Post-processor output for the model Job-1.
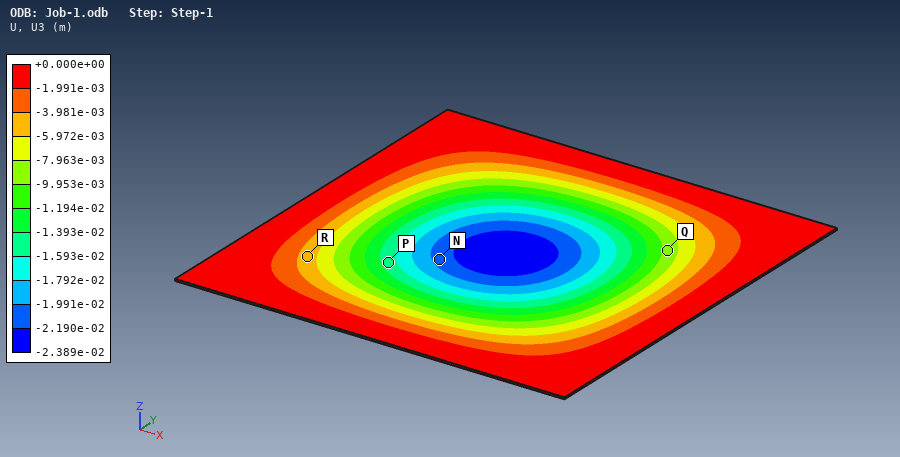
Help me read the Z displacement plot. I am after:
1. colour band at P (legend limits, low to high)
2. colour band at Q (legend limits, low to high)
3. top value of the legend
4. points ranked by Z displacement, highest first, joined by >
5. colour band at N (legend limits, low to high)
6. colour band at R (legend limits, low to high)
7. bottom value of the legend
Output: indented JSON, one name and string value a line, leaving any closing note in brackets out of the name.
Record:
{
  "colour band at P": "-1.593e-02 to -1.393e-02 m",
  "colour band at Q": "-9.953e-03 to -7.963e-03 m",
  "top value of the legend": "+0.000e+00 m",
  "points ranked by Z displacement, highest first, joined by >": "R > Q > P > N",
  "colour band at N": "-2.190e-02 to -1.991e-02 m",
  "colour band at R": "-5.972e-03 to -3.981e-03 m",
  "bottom value of the legend": "-2.389e-02 m"
}
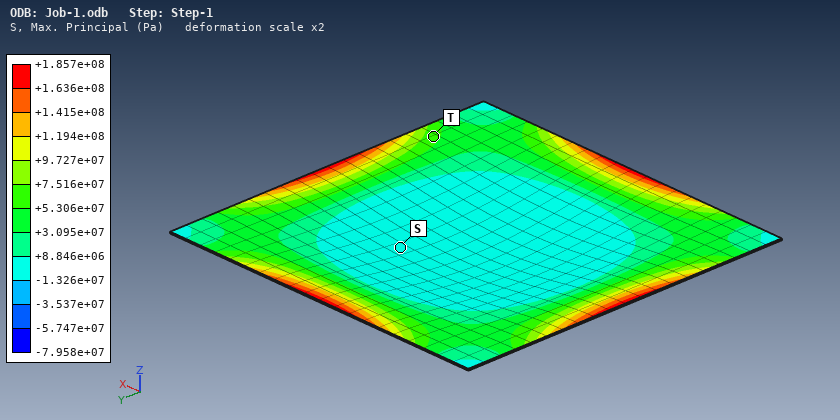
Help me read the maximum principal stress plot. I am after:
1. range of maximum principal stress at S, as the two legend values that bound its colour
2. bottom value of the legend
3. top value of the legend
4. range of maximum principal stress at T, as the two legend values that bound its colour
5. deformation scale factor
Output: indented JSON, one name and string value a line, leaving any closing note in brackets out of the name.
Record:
{
  "range of maximum principal stress at S, as the two legend values that bound its colour": "-1.326e+07 to +8.846e+06 Pa",
  "bottom value of the legend": "-7.958e+07 Pa",
  "top value of the legend": "+1.857e+08 Pa",
  "range of maximum principal stress at T, as the two legend values that bound its colour": "+5.306e+07 to +7.516e+07 Pa",
  "deformation scale factor": "2"
}
